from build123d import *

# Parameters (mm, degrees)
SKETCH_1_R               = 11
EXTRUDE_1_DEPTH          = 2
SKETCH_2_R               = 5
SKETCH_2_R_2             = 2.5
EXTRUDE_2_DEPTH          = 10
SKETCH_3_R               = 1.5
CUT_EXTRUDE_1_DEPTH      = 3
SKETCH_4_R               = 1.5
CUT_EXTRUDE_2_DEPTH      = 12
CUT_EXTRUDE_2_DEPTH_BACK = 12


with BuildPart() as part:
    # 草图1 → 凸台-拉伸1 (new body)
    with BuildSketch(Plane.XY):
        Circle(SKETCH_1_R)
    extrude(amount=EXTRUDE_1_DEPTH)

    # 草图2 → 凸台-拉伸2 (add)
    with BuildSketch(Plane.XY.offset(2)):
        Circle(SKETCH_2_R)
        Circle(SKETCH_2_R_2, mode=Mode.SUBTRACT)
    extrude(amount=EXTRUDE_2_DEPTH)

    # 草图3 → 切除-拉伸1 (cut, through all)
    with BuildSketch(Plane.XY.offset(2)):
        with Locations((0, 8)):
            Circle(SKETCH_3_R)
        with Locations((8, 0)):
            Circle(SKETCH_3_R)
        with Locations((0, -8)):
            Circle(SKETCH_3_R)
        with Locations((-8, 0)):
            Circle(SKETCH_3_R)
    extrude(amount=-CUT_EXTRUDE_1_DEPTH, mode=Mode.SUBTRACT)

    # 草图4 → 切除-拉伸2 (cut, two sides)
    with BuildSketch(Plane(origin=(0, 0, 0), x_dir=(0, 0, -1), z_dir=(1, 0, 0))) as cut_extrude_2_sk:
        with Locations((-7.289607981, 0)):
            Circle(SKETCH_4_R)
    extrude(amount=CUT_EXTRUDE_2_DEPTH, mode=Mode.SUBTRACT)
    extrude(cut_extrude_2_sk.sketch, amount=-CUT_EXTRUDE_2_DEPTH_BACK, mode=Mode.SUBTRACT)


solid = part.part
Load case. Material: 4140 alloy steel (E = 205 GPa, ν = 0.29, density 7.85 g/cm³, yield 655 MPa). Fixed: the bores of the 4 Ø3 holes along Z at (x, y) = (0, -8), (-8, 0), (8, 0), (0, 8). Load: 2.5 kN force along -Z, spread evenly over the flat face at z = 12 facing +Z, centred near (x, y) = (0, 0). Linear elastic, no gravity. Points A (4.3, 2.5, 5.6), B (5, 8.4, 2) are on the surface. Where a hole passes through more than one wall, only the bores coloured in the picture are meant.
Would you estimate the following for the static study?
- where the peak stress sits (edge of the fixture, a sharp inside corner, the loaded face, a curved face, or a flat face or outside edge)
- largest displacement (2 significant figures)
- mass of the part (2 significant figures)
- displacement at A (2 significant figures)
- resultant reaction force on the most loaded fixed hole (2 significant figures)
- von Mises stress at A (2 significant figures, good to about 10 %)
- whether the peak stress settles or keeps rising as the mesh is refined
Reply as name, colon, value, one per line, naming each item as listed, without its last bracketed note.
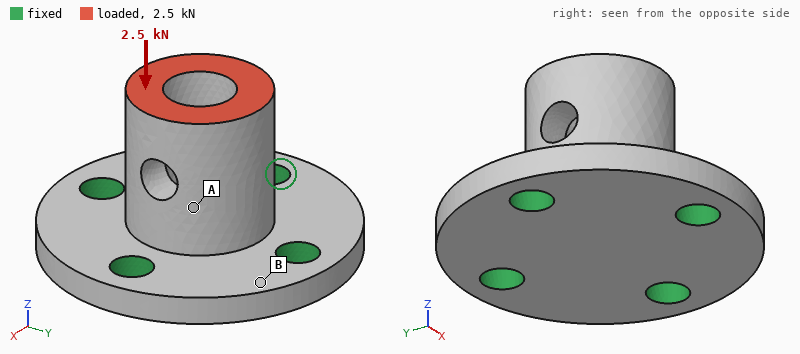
where the peak stress sits: edge of the fixture
largest displacement: 6.7 µm
mass of the part: 9.9 g
displacement at A: 4.5 µm
resultant reaction force on the most loaded fixed hole: 670 N
von Mises stress at A: 64 MPa
whether the peak stress settles or keeps rising as the mesh is refined: keeps rising
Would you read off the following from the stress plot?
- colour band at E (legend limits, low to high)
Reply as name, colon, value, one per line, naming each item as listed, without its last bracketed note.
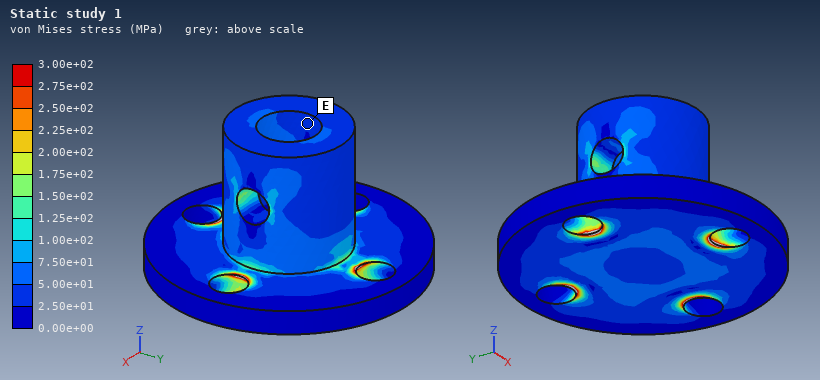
colour band at E: 2.50e+01 to 5.00e+01 MPa
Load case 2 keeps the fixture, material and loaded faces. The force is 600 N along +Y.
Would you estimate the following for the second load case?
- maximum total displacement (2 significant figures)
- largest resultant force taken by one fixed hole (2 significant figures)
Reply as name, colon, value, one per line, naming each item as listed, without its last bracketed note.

maximum total displacement: 12 µm
largest resultant force taken by one fixed hole: 540 N
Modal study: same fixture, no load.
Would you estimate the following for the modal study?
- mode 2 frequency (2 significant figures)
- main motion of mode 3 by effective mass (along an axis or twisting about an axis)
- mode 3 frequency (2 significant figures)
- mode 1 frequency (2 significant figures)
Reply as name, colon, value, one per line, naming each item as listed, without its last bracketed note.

mode 2 frequency: 30 kHz
main motion of mode 3 by effective mass: along Z
mode 3 frequency: 50 kHz
mode 1 frequency: 29 kHz
